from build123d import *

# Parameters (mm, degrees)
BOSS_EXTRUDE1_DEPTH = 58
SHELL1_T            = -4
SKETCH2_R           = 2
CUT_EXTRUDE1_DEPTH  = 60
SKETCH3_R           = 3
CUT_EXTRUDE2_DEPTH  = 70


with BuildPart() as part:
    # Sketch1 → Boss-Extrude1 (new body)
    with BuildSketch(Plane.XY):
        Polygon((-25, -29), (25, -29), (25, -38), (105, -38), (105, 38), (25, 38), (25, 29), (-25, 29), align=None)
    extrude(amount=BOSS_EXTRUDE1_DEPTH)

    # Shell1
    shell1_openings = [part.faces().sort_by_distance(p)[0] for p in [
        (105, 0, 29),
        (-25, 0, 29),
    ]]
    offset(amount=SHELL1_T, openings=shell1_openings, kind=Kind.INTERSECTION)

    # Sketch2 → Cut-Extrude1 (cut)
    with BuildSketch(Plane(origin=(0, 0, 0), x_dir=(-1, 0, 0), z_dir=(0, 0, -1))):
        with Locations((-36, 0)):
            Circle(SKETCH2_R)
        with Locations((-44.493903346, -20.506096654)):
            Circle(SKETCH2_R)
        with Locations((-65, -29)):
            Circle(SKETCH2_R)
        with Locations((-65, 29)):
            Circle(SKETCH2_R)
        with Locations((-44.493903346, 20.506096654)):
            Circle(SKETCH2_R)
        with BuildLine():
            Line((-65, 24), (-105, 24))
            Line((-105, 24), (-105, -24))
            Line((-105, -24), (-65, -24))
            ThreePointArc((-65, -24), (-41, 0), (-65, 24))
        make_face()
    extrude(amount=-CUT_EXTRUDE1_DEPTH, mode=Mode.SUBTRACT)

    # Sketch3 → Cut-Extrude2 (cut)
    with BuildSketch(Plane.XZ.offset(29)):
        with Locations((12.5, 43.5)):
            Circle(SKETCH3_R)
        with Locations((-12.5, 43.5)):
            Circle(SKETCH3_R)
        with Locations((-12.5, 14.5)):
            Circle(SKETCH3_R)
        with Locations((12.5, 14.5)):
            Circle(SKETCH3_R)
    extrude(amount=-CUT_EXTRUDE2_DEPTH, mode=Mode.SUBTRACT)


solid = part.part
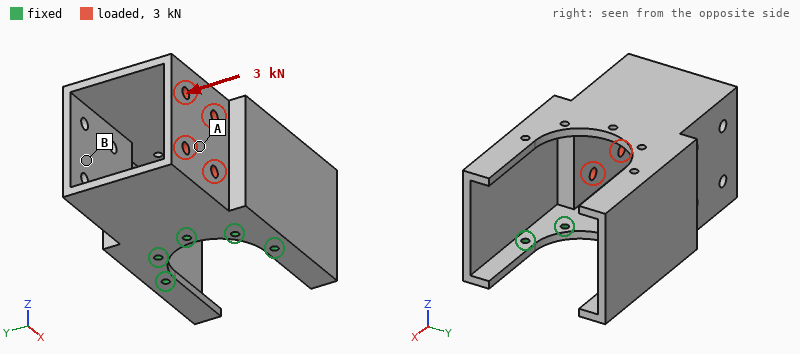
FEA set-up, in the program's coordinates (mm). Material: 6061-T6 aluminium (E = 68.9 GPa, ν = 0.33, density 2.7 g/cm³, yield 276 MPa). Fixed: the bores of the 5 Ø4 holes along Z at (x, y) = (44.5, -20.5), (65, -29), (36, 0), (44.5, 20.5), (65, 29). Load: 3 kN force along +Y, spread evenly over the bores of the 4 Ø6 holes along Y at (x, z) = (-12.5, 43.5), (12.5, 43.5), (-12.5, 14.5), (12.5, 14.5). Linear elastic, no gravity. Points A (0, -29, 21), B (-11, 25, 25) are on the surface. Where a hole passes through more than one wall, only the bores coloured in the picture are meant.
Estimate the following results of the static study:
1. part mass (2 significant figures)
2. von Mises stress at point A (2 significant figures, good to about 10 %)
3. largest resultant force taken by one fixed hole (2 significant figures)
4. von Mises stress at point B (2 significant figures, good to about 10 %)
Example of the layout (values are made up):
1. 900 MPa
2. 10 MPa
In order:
1. 280 g
2. 35 MPa
3. 1.7 kN
4. 15 MPa
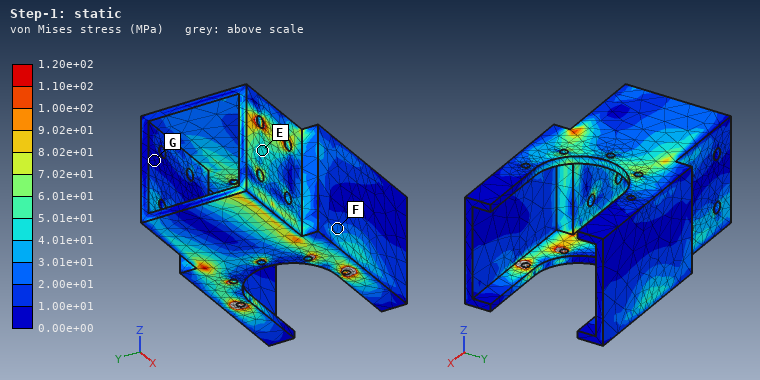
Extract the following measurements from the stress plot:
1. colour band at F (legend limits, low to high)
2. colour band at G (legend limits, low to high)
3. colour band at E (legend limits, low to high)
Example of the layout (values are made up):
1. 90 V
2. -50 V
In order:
1. 2.00e+01 to 3.01e+01 MPa
2. 0.00e+00 to 1.00e+01 MPa
3. 4.01e+01 to 5.01e+01 MPa
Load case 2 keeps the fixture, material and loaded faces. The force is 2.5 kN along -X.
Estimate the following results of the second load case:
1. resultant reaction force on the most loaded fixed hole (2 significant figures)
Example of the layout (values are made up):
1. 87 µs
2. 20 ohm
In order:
1. 1.8 kN
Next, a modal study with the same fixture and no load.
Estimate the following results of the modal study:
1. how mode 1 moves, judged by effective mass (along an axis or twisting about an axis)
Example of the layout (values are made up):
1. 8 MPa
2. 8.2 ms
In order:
1. along Y
